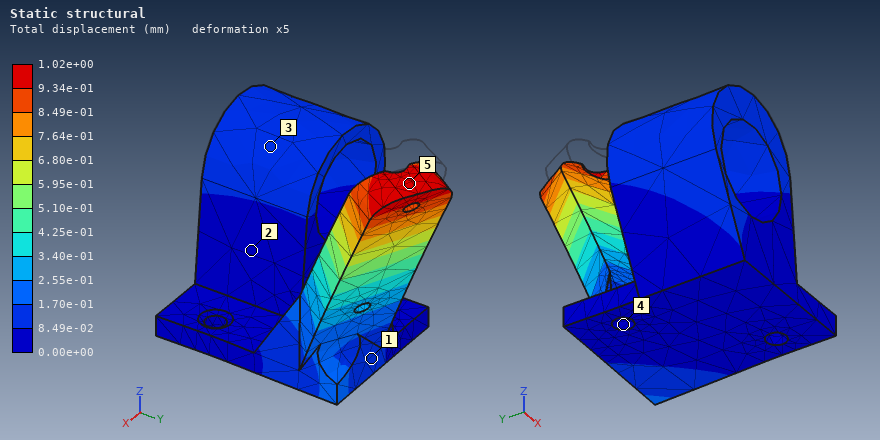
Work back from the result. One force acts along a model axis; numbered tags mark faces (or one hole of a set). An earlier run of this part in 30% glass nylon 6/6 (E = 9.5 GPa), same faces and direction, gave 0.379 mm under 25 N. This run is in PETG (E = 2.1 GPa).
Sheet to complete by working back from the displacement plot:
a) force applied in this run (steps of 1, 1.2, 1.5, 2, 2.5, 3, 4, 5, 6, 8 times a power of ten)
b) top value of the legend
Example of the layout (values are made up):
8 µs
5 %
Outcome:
15 N
1.02e+00 mm
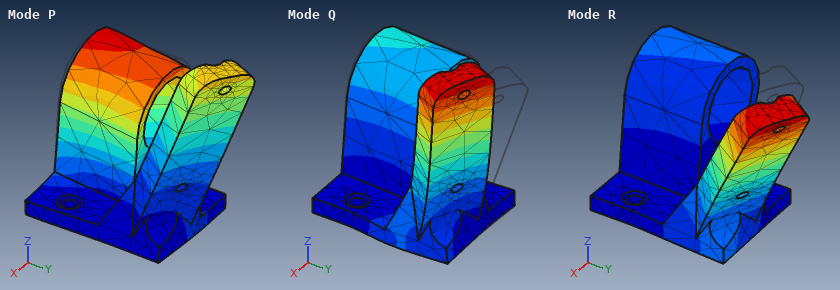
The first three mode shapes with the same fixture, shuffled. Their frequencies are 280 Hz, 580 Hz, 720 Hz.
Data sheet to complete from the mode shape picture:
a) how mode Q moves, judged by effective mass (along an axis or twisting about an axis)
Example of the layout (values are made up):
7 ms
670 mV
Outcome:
along X
